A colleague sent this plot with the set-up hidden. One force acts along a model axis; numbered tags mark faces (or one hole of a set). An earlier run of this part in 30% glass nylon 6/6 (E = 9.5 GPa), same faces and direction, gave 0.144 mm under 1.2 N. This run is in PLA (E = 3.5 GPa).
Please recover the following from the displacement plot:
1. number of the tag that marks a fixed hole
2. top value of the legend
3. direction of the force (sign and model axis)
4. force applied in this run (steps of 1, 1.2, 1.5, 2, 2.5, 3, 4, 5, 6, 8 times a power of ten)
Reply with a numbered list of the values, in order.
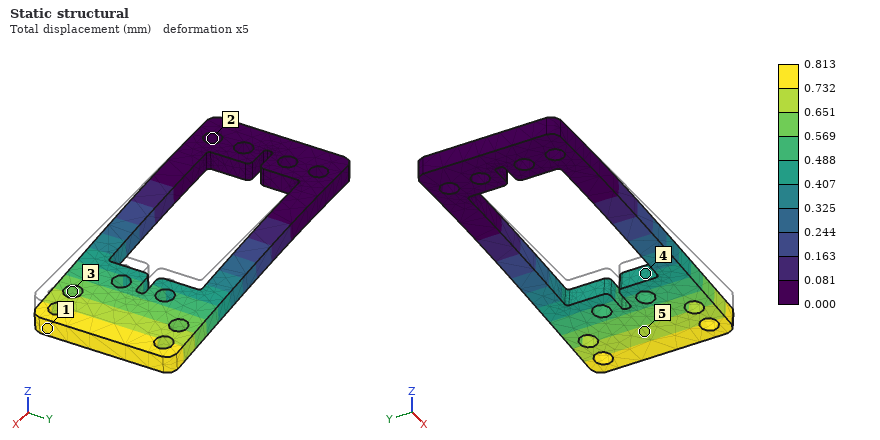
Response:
1. 2
2. 0.813 mm
3. -Z
4. 2.5 N
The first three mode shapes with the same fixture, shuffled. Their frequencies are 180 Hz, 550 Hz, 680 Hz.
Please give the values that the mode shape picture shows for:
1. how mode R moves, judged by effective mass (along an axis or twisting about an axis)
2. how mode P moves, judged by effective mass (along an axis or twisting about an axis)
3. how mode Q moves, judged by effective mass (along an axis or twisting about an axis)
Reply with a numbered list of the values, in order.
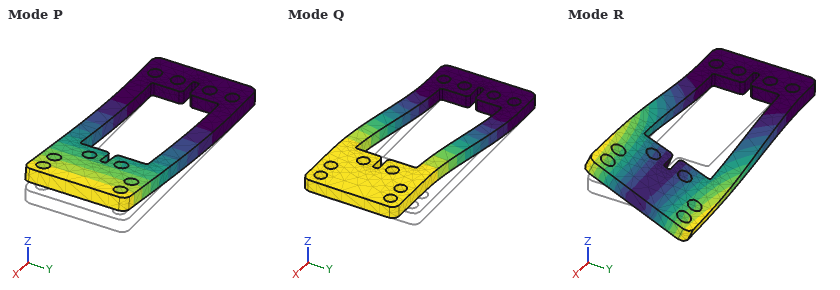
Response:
1. twisting about X
2. along Z
3. along Y
